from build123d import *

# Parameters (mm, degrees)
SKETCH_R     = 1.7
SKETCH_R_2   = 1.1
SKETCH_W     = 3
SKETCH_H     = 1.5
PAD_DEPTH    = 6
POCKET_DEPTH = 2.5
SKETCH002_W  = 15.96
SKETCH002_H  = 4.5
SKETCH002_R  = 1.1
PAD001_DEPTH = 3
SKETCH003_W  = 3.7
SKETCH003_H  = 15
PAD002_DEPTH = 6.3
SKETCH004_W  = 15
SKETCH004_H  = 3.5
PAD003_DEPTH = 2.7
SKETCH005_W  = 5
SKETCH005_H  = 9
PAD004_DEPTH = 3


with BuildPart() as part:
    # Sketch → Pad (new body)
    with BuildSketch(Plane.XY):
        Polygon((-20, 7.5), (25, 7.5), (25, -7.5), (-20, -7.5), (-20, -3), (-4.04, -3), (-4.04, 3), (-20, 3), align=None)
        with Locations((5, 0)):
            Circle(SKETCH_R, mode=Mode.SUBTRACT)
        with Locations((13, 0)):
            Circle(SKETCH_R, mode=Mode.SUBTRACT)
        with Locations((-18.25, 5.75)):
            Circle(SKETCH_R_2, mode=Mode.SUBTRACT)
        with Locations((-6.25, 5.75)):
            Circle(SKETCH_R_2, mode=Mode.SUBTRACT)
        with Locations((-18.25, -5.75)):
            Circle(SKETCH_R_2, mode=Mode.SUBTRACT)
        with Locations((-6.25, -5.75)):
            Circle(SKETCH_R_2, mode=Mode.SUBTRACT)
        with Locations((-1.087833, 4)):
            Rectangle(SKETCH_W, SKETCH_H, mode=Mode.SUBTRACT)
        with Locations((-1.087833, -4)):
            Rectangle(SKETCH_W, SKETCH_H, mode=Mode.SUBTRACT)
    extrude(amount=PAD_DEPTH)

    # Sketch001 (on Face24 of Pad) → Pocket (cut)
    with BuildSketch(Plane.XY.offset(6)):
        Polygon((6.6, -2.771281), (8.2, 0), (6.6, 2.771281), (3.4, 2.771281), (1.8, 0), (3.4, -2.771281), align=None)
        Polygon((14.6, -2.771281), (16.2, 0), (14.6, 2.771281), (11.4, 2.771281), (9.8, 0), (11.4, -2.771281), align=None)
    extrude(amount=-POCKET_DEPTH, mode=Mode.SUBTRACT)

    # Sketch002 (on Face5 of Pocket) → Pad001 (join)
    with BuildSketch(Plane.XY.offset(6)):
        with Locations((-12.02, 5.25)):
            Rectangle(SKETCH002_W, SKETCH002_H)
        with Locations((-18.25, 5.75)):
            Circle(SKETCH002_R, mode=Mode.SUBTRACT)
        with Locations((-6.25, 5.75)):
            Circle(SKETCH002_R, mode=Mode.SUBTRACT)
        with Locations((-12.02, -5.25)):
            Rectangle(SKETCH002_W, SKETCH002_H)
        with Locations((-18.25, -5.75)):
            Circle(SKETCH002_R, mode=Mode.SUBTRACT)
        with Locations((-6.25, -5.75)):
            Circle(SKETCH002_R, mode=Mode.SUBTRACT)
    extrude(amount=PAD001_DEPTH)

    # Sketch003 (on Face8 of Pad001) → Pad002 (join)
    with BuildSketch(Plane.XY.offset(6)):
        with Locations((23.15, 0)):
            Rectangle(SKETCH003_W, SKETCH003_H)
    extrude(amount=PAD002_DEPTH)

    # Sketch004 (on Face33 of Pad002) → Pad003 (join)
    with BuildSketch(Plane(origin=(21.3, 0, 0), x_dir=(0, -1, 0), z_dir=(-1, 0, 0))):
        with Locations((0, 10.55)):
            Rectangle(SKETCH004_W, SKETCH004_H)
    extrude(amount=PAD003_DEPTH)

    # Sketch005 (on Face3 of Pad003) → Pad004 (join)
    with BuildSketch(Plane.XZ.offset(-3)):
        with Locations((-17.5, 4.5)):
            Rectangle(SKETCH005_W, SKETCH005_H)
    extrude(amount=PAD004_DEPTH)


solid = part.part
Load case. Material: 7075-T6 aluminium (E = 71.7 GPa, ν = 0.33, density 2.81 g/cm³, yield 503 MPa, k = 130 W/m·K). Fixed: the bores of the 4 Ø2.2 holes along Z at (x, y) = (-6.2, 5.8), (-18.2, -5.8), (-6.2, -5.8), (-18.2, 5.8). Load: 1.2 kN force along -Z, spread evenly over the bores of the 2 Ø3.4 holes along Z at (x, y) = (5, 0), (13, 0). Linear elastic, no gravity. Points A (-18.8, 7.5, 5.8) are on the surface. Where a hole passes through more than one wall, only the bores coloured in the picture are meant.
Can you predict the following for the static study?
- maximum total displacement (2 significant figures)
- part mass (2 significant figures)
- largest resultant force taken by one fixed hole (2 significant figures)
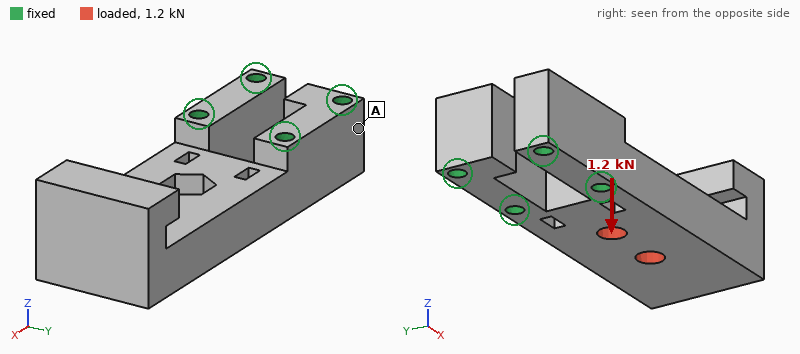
0.31 mm
12 g
630 N
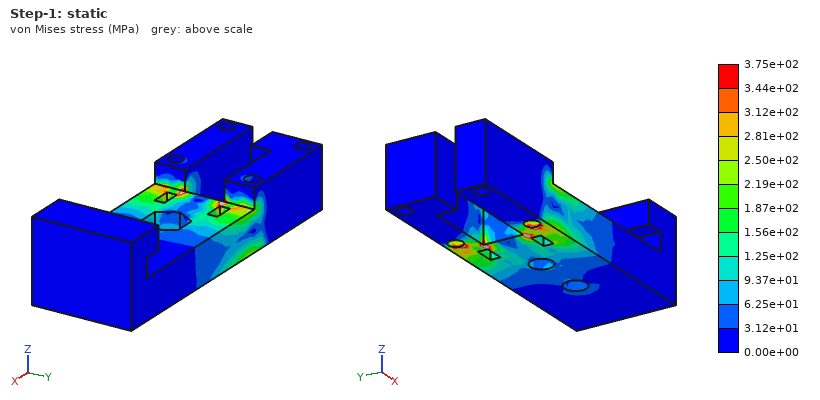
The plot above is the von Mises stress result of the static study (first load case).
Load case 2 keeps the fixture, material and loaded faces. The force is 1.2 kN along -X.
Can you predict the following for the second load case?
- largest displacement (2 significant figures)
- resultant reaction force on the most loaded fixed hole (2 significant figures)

39 µm
600 N
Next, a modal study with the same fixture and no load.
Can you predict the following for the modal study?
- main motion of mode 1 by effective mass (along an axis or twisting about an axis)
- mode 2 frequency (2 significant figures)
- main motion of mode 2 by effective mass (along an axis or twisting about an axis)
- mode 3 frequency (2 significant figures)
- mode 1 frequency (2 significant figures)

along Z
7500 Hz
along Y
12 kHz
3300 Hz
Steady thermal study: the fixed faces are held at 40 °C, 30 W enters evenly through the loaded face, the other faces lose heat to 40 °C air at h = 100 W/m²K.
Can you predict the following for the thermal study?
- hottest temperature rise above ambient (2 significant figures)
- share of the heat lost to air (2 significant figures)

45 K
20 %
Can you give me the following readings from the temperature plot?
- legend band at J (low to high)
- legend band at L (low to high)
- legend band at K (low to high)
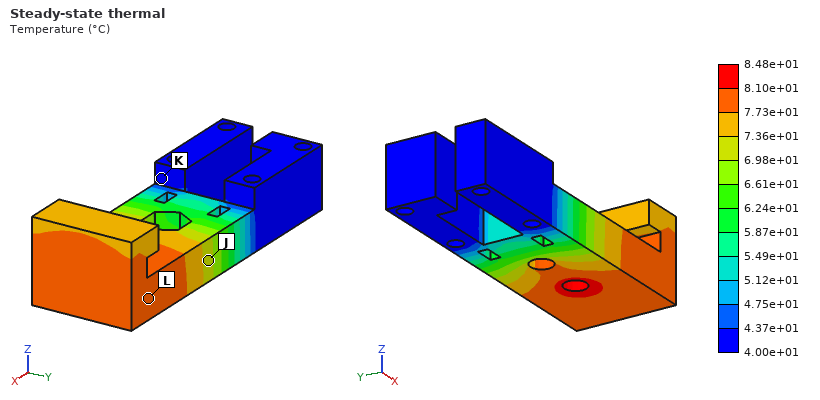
6.98e+01 to 7.36e+01 °C
7.73e+01 to 8.10e+01 °C
4.00e+01 to 4.37e+01 °C
